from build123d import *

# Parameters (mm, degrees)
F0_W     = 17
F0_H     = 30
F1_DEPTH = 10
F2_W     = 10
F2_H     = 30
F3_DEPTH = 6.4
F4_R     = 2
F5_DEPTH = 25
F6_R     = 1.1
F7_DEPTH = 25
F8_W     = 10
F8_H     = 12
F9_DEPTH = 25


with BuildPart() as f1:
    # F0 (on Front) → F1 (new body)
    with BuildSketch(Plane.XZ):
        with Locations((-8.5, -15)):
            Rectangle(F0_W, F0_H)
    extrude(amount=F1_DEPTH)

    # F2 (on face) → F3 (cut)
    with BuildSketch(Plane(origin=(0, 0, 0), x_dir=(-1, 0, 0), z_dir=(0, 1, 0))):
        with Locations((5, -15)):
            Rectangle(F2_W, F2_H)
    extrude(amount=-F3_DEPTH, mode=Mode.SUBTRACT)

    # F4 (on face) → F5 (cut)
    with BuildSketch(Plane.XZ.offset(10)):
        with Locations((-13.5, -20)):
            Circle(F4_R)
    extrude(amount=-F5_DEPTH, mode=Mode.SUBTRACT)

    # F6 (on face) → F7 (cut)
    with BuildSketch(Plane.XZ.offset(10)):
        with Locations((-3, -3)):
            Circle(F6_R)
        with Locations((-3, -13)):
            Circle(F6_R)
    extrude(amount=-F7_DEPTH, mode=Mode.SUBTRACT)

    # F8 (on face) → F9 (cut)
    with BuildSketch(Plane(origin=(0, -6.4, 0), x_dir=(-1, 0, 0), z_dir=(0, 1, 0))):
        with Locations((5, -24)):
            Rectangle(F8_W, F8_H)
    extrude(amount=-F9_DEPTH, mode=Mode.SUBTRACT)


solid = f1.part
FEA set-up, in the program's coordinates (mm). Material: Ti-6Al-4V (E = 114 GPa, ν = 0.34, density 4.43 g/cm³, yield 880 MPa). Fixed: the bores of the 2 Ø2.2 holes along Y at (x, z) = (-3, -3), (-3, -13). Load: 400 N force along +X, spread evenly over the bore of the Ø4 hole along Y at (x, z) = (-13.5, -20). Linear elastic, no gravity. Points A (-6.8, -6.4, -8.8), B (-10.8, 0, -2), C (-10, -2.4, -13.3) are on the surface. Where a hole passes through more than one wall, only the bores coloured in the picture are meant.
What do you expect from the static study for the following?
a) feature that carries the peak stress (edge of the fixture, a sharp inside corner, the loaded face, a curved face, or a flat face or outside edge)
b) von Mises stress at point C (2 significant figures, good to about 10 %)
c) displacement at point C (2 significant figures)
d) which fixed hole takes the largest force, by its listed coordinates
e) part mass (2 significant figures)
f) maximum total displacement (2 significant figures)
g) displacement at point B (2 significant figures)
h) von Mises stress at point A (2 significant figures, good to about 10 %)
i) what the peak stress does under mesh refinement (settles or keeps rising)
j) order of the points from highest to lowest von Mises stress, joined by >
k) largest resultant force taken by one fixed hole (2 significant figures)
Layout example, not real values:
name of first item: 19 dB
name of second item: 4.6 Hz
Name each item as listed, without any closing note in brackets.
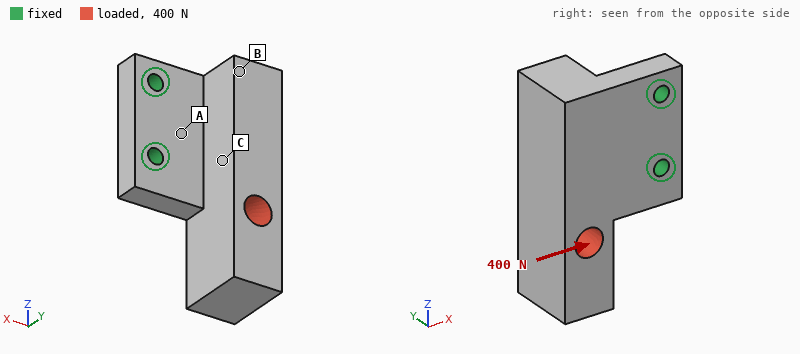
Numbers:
feature that carries the peak stress: edge of the fixture
von Mises stress at point C: 15 MPa
displacement at point C: 11 µm
which fixed hole takes the largest force, by its listed coordinates: (-3, -13)
part mass: 11 g
maximum total displacement: 32 µm
displacement at point B: 9.5 µm
von Mises stress at point A: 29 MPa
what the peak stress does under mesh refinement: keeps rising
order of the points from highest to lowest von Mises stress, joined by >: A > C > B
largest resultant force taken by one fixed hole: 630 N
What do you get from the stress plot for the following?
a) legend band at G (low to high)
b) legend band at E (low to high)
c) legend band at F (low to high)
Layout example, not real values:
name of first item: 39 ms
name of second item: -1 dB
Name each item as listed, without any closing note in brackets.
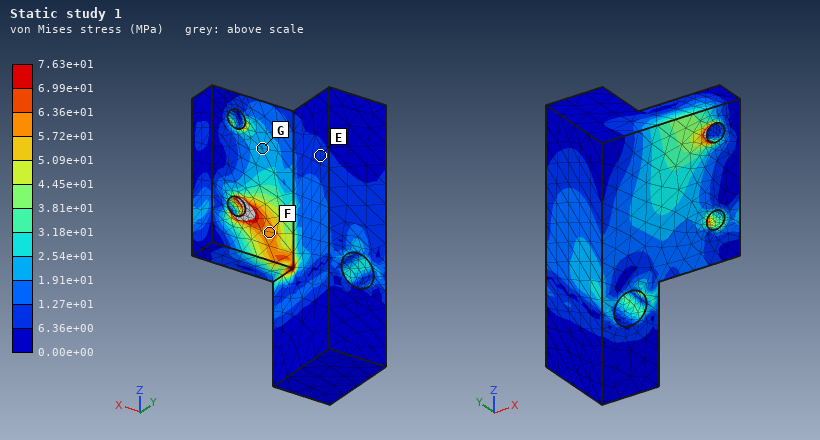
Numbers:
legend band at G: 1.91e+01 to 2.54e+01 MPa
legend band at E: 6.36e+00 to 1.27e+01 MPa
legend band at F: 5.72e+01 to 6.36e+01 MPa
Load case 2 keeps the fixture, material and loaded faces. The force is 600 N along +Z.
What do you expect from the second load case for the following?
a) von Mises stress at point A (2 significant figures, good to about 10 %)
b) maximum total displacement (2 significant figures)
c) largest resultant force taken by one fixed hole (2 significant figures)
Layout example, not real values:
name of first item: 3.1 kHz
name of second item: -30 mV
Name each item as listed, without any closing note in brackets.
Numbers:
von Mises stress at point A: 42 MPa
maximum total displacement: 18 µm
largest resultant force taken by one fixed hole: 630 N
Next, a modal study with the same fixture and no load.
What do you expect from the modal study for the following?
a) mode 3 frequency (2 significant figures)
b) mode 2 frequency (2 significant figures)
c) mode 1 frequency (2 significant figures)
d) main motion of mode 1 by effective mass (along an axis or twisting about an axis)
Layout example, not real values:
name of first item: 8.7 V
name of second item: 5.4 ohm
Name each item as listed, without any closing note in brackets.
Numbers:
mode 3 frequency: 12 kHz
mode 2 frequency: 9400 Hz
mode 1 frequency: 5500 Hz
main motion of mode 1 by effective mass: along Y
